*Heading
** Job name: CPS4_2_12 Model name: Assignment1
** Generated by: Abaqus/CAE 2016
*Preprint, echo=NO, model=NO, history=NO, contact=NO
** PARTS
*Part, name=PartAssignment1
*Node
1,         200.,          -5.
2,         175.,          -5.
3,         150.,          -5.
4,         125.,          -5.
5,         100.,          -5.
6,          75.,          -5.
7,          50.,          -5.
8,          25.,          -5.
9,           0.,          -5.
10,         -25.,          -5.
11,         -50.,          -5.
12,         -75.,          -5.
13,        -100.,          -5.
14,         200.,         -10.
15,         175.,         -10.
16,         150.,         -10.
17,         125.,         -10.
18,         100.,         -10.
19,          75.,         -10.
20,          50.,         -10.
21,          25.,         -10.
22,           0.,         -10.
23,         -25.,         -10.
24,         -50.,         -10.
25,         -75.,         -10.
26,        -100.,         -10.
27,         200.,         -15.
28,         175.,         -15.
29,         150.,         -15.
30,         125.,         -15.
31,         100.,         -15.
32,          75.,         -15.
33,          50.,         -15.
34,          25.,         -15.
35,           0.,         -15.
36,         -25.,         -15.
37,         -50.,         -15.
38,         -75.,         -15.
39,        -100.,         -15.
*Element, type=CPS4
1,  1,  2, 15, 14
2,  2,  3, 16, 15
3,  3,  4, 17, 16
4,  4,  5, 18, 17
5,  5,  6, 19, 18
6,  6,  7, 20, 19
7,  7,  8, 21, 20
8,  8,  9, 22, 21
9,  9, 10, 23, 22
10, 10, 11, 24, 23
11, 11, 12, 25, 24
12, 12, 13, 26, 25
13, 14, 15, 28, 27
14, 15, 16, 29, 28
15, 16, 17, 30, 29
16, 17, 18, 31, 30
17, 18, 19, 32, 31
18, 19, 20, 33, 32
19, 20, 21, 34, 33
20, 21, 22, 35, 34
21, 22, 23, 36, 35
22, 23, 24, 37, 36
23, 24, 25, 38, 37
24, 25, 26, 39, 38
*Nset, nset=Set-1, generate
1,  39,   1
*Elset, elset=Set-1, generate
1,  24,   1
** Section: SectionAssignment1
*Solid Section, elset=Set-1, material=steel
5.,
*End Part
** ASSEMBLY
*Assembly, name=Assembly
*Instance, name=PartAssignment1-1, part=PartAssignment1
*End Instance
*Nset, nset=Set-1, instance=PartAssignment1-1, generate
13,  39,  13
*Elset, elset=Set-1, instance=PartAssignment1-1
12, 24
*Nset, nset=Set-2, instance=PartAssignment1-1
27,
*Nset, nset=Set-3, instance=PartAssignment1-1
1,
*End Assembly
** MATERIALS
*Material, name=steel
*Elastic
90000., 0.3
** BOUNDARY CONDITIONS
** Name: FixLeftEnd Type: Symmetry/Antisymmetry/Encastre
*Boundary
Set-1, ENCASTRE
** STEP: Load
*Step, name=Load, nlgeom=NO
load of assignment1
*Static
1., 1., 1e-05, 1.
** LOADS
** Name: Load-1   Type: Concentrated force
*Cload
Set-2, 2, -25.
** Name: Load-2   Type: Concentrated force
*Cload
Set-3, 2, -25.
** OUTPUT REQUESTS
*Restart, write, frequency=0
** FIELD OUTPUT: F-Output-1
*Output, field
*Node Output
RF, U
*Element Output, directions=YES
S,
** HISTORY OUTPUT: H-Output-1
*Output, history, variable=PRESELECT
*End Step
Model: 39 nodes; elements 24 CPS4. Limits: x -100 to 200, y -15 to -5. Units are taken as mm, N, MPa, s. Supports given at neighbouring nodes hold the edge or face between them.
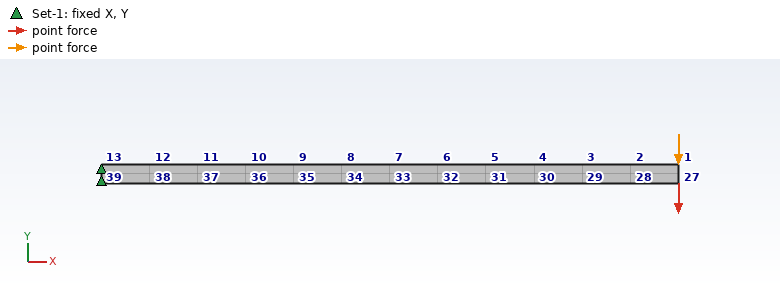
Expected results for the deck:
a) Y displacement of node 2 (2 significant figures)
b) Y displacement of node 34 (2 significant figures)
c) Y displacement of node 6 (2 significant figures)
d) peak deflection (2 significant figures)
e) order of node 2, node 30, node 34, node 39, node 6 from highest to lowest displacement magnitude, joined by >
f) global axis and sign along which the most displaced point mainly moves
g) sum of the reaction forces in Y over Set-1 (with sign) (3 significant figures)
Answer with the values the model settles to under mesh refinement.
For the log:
-10 mm
-2.7 mm
-4.9 mm
12 mm
node 2 > node 30 > node 6 > node 34 > node 39
-Y
50.0 N
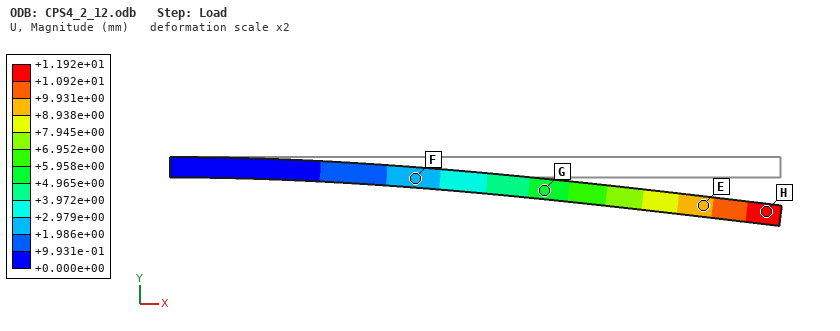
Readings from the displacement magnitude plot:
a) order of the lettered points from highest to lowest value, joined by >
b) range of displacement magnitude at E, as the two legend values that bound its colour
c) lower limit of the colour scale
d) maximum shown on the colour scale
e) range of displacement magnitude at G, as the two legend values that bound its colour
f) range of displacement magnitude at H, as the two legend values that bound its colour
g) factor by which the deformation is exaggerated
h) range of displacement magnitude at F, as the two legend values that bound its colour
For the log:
H > E > G > F
+8.938e+00 to +9.931e+00 mm
+0.000e+00 mm
+1.192e+01 mm
+4.965e+00 to +5.958e+00 mm
+1.092e+01 to +1.192e+01 mm
2
+1.986e+00 to +2.979e+00 mm
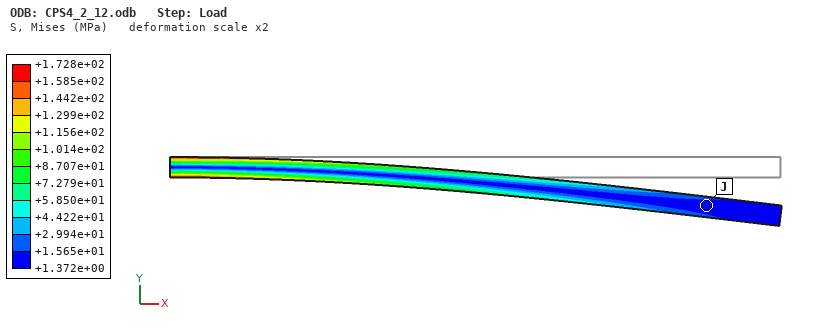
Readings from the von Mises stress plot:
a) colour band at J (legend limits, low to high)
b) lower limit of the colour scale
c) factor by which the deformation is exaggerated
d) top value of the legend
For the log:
+1.372e+00 to +1.565e+01 MPa
+1.372e+00 MPa
2
+1.728e+02 MPa
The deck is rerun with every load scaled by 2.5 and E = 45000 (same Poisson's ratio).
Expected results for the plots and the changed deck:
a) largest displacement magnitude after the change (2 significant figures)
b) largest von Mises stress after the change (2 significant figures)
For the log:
60 mm
430 MPa
